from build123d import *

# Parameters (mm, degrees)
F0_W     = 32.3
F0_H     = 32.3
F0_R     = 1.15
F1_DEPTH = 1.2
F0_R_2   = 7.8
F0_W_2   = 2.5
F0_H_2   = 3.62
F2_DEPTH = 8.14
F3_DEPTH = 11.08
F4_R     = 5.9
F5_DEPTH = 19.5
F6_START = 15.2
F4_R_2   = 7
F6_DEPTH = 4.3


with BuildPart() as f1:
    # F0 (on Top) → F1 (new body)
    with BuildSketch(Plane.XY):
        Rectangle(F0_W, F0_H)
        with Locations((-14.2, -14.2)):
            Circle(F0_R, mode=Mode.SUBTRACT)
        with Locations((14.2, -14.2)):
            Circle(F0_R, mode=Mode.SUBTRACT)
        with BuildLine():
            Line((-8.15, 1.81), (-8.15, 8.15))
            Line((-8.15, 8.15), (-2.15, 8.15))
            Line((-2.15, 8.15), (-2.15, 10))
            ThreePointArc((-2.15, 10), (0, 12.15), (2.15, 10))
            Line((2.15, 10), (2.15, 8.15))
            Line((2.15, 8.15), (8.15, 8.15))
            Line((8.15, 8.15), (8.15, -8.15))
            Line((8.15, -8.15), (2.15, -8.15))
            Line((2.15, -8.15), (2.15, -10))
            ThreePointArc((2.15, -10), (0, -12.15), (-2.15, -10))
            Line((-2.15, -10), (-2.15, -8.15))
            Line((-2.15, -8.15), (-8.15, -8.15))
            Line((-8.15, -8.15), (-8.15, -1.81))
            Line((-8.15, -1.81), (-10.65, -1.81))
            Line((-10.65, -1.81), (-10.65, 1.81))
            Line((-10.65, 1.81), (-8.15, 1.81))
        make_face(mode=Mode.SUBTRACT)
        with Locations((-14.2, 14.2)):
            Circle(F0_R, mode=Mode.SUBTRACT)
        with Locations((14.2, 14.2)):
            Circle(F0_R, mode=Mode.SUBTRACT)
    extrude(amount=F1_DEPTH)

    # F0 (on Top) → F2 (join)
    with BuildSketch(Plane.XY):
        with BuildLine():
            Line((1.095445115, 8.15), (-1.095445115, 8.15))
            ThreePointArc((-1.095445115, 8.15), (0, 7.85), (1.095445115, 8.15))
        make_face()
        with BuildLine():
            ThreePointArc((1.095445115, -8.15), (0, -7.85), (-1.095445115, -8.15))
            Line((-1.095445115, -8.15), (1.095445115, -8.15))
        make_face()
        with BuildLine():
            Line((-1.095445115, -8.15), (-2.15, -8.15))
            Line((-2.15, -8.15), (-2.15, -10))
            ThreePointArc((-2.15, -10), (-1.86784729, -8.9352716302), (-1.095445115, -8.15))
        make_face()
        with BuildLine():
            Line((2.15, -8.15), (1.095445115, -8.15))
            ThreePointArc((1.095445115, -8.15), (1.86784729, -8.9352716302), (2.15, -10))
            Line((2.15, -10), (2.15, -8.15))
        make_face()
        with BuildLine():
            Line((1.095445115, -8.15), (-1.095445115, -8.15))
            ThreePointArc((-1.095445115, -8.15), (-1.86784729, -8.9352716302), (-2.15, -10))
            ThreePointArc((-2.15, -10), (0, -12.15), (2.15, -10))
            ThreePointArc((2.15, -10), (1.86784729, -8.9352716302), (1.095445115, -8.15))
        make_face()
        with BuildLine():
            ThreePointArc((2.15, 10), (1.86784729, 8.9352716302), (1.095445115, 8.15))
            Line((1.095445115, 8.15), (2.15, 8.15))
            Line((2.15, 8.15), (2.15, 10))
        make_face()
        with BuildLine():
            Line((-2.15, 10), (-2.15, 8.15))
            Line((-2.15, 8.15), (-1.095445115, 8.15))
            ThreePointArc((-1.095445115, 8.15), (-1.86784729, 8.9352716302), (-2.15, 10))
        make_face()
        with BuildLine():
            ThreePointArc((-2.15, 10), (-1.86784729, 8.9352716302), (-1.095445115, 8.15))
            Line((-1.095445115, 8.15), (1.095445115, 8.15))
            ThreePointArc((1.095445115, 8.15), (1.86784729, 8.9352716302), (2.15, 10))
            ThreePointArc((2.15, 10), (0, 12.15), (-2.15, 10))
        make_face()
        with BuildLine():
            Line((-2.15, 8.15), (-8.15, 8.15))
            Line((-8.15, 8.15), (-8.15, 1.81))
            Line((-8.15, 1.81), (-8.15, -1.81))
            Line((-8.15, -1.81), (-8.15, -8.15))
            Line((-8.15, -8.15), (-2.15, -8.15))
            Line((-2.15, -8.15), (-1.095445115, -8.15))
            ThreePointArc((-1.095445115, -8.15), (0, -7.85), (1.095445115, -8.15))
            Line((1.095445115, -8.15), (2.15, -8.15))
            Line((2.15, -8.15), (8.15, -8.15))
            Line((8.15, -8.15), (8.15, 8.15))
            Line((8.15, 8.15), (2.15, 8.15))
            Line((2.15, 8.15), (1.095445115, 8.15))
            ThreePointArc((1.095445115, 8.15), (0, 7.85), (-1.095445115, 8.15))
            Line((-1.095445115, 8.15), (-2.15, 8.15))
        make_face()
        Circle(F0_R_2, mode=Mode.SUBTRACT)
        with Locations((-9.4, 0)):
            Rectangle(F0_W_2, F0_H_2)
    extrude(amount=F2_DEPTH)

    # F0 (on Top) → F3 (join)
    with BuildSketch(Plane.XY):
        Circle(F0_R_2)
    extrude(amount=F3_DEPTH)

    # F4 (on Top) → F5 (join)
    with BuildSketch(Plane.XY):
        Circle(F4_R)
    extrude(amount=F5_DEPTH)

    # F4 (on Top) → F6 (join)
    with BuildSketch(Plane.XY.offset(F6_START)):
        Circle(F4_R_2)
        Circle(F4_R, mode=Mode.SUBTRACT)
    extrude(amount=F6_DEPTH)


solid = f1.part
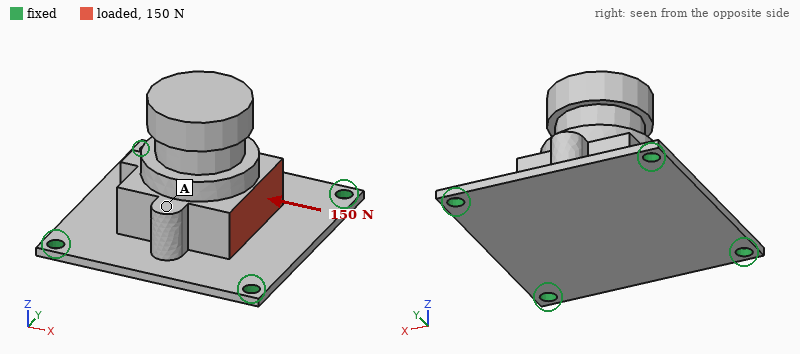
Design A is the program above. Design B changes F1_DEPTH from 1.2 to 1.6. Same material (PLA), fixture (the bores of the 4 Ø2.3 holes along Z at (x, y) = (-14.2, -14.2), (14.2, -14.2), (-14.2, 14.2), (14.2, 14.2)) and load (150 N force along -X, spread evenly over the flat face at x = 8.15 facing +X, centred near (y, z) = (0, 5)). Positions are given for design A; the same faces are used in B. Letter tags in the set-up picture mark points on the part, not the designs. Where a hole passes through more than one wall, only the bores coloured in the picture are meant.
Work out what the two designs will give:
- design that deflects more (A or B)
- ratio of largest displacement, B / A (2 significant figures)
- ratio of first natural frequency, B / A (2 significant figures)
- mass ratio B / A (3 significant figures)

A
0.50
1.4
1.06
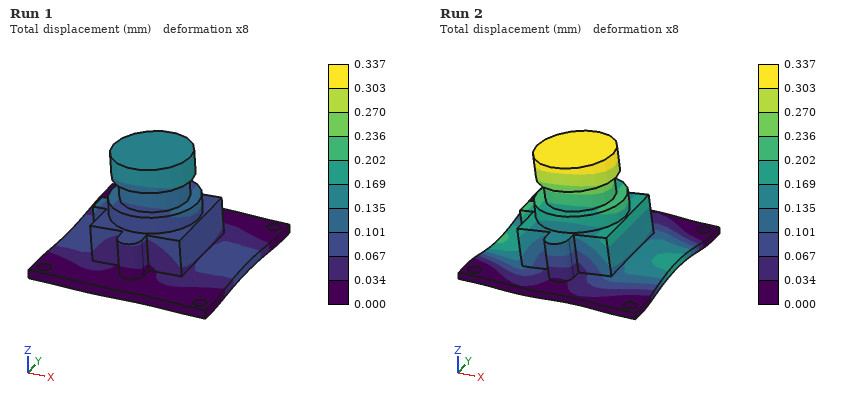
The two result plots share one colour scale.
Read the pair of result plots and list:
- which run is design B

Run 1
